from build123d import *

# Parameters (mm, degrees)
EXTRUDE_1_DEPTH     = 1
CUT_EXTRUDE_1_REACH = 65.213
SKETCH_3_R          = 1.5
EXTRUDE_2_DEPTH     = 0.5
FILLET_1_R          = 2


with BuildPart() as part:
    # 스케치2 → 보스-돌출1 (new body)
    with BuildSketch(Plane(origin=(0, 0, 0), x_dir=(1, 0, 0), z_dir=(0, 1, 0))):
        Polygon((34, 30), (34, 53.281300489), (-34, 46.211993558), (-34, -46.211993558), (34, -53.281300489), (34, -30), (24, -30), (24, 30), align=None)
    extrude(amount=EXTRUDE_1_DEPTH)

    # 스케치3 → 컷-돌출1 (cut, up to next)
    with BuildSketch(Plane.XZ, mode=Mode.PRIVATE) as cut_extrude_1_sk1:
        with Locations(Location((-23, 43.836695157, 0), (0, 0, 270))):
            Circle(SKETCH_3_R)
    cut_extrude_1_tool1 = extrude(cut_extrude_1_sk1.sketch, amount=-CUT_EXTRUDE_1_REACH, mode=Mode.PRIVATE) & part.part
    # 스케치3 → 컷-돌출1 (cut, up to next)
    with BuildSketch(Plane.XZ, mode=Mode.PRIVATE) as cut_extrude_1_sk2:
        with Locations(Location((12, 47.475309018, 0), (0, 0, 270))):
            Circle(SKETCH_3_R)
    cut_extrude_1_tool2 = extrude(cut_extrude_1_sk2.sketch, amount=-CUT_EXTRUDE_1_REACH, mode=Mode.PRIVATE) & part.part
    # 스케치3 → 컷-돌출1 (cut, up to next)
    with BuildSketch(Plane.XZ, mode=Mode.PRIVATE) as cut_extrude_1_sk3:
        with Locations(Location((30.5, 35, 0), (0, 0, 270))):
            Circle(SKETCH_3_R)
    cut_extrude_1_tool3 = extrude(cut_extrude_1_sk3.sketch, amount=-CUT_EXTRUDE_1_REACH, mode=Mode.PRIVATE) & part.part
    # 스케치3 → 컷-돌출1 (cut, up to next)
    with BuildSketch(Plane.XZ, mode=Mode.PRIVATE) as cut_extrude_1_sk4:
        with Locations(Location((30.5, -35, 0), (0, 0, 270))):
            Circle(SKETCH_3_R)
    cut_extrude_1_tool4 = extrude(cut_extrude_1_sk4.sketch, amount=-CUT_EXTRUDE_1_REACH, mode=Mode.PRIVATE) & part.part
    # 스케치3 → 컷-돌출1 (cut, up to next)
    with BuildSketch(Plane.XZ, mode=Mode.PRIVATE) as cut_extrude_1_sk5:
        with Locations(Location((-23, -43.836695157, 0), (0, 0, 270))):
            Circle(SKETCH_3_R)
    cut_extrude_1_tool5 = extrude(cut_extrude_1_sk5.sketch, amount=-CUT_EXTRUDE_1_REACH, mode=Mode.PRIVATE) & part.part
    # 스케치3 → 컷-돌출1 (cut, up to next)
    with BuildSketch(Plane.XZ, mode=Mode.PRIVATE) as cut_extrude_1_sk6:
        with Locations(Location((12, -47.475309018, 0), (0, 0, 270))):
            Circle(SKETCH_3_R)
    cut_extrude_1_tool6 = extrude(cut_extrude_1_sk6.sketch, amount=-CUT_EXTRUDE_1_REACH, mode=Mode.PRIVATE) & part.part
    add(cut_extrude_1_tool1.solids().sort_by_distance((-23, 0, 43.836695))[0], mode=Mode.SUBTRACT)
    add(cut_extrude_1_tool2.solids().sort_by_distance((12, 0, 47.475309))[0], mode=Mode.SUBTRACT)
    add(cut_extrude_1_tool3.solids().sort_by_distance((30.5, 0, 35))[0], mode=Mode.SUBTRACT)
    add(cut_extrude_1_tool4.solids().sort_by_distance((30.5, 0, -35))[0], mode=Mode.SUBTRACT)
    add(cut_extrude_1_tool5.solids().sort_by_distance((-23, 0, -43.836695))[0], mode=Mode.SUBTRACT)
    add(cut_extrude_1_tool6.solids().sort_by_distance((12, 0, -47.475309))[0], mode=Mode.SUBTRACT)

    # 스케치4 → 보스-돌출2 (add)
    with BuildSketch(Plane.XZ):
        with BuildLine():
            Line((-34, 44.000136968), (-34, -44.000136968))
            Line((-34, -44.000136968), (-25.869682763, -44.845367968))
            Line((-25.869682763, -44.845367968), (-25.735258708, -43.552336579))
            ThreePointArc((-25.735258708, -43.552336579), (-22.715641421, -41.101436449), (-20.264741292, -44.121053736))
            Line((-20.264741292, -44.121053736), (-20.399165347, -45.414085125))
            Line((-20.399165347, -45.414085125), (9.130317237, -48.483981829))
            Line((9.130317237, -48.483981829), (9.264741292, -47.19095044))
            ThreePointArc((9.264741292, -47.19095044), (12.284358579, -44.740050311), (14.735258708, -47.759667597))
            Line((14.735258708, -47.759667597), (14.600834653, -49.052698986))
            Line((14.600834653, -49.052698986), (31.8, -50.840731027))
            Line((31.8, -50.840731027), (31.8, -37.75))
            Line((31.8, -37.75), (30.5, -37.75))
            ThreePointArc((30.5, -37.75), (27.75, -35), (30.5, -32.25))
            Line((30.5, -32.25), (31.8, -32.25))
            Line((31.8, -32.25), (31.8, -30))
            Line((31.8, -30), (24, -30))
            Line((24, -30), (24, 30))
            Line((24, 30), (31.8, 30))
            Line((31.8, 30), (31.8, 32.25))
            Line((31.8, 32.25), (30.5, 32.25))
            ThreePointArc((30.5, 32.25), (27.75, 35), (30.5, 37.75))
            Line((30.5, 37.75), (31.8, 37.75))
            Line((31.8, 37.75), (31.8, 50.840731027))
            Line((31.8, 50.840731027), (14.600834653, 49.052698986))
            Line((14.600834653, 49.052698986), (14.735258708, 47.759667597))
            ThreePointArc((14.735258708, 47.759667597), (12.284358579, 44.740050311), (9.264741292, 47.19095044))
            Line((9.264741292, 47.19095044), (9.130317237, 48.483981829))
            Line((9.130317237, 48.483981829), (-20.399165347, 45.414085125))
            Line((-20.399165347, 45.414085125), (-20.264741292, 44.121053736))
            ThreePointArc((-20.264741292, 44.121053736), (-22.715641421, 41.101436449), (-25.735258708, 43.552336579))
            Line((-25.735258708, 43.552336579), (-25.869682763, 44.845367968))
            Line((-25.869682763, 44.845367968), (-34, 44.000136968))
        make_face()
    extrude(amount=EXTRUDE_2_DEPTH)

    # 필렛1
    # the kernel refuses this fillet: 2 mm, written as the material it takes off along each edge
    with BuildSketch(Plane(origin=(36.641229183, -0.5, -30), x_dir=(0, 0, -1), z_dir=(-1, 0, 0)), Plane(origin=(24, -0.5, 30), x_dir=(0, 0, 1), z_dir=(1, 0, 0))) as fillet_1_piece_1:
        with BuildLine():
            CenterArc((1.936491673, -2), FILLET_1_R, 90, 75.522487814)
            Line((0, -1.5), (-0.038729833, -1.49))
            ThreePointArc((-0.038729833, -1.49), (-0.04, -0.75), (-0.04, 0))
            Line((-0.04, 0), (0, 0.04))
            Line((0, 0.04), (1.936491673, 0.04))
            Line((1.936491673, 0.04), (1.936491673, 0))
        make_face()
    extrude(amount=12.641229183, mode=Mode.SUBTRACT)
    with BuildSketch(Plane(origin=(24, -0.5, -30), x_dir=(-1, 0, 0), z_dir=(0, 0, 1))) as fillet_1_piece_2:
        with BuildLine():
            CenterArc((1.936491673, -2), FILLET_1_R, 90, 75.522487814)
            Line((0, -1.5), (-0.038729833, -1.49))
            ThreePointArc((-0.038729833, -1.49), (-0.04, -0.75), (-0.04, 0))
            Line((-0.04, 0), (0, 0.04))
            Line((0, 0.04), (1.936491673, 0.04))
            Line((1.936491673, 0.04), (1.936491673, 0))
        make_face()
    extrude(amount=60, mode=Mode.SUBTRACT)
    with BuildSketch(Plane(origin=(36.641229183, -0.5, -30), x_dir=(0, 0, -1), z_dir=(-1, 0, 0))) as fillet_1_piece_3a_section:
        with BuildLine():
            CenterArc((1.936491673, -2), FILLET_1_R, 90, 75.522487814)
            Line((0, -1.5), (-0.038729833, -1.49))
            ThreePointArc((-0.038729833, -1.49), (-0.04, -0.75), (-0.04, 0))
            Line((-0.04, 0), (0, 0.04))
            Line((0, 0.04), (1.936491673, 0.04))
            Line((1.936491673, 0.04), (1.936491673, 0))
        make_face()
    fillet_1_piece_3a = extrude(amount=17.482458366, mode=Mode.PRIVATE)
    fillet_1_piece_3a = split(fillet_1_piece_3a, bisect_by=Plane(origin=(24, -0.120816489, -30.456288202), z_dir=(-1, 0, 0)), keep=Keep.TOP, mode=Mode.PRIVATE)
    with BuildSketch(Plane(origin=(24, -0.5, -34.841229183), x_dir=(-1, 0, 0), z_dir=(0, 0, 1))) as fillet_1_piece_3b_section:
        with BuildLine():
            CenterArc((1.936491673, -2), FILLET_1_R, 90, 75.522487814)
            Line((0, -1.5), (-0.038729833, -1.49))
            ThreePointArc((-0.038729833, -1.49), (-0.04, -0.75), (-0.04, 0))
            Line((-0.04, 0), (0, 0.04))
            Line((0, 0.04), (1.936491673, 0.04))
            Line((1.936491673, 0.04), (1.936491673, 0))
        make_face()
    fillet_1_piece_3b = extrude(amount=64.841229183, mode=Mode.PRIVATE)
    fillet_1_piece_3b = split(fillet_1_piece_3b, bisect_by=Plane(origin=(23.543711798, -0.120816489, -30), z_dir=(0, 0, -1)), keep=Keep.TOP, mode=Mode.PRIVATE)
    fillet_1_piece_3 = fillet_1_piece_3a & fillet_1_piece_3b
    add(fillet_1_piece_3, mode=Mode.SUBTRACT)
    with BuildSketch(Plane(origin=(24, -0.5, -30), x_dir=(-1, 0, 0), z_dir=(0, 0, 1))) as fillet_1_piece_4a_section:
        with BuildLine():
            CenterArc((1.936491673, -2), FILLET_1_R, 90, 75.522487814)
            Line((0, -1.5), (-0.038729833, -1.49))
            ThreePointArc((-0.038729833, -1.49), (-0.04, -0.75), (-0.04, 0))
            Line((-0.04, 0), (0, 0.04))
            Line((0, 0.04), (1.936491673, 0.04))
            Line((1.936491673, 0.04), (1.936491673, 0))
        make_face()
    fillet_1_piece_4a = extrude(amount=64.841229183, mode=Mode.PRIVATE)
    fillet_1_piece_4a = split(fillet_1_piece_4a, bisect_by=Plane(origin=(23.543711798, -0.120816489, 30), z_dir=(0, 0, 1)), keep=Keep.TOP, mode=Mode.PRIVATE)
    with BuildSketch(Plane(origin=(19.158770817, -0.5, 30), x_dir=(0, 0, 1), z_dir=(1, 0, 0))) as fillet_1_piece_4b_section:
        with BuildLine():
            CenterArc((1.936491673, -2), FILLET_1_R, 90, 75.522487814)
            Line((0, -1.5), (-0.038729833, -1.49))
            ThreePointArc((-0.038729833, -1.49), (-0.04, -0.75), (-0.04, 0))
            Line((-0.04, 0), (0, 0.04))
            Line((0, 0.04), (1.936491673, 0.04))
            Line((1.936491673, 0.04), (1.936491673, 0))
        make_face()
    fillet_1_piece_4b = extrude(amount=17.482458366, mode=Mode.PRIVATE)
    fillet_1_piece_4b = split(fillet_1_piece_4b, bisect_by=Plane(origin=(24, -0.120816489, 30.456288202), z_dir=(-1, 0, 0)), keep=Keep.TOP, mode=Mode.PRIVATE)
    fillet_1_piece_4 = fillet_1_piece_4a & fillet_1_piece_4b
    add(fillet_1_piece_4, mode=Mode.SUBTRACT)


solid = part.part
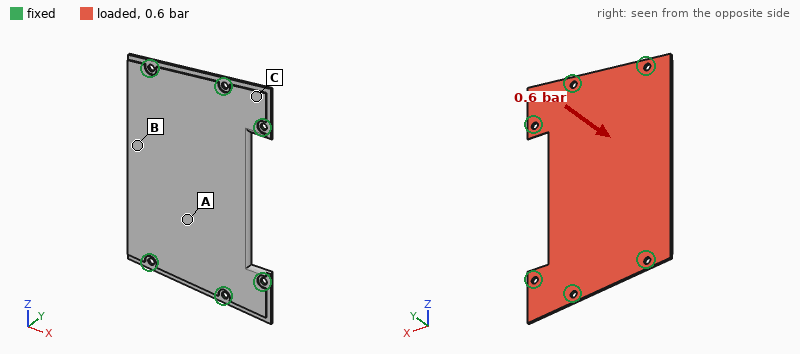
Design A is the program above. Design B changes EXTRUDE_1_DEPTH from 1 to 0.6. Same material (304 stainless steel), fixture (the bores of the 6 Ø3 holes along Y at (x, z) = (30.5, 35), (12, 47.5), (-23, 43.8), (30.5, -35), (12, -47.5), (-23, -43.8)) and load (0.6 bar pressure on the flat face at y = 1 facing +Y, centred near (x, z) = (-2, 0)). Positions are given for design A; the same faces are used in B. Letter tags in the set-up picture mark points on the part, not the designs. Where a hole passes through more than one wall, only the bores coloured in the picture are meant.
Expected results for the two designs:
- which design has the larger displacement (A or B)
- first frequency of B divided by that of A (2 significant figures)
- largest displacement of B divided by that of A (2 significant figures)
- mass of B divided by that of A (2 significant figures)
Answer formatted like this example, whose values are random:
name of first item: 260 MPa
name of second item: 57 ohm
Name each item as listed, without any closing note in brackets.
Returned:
which design has the larger displacement: B
first frequency of B divided by that of A: 0.71
largest displacement of B divided by that of A: 2.7
mass of B divided by that of A: 0.72
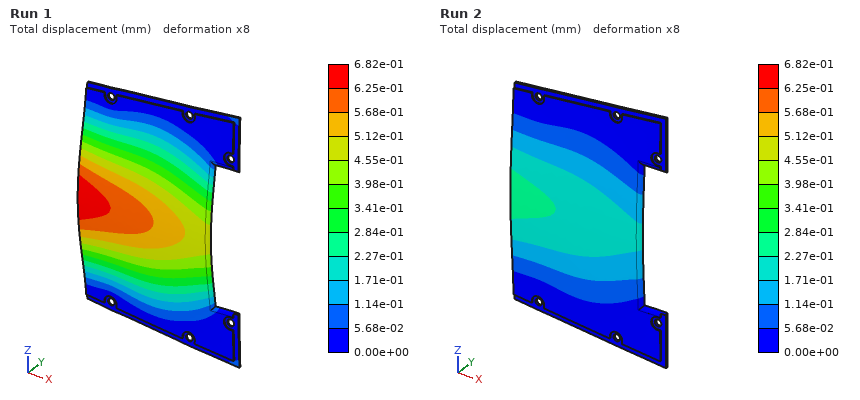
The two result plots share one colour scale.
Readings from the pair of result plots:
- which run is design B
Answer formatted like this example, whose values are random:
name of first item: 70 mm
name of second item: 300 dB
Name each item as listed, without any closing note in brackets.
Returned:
which run is design B: Run 1
